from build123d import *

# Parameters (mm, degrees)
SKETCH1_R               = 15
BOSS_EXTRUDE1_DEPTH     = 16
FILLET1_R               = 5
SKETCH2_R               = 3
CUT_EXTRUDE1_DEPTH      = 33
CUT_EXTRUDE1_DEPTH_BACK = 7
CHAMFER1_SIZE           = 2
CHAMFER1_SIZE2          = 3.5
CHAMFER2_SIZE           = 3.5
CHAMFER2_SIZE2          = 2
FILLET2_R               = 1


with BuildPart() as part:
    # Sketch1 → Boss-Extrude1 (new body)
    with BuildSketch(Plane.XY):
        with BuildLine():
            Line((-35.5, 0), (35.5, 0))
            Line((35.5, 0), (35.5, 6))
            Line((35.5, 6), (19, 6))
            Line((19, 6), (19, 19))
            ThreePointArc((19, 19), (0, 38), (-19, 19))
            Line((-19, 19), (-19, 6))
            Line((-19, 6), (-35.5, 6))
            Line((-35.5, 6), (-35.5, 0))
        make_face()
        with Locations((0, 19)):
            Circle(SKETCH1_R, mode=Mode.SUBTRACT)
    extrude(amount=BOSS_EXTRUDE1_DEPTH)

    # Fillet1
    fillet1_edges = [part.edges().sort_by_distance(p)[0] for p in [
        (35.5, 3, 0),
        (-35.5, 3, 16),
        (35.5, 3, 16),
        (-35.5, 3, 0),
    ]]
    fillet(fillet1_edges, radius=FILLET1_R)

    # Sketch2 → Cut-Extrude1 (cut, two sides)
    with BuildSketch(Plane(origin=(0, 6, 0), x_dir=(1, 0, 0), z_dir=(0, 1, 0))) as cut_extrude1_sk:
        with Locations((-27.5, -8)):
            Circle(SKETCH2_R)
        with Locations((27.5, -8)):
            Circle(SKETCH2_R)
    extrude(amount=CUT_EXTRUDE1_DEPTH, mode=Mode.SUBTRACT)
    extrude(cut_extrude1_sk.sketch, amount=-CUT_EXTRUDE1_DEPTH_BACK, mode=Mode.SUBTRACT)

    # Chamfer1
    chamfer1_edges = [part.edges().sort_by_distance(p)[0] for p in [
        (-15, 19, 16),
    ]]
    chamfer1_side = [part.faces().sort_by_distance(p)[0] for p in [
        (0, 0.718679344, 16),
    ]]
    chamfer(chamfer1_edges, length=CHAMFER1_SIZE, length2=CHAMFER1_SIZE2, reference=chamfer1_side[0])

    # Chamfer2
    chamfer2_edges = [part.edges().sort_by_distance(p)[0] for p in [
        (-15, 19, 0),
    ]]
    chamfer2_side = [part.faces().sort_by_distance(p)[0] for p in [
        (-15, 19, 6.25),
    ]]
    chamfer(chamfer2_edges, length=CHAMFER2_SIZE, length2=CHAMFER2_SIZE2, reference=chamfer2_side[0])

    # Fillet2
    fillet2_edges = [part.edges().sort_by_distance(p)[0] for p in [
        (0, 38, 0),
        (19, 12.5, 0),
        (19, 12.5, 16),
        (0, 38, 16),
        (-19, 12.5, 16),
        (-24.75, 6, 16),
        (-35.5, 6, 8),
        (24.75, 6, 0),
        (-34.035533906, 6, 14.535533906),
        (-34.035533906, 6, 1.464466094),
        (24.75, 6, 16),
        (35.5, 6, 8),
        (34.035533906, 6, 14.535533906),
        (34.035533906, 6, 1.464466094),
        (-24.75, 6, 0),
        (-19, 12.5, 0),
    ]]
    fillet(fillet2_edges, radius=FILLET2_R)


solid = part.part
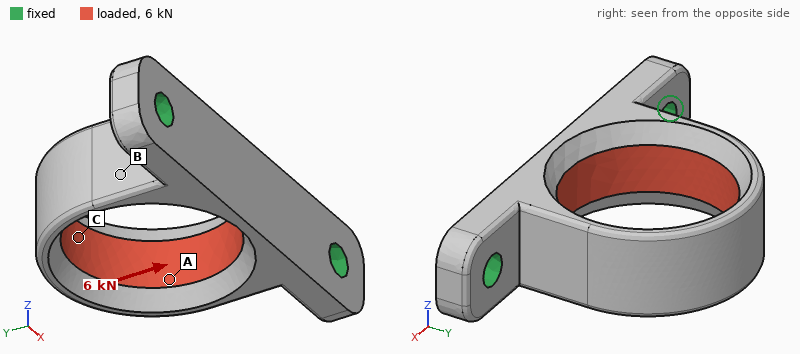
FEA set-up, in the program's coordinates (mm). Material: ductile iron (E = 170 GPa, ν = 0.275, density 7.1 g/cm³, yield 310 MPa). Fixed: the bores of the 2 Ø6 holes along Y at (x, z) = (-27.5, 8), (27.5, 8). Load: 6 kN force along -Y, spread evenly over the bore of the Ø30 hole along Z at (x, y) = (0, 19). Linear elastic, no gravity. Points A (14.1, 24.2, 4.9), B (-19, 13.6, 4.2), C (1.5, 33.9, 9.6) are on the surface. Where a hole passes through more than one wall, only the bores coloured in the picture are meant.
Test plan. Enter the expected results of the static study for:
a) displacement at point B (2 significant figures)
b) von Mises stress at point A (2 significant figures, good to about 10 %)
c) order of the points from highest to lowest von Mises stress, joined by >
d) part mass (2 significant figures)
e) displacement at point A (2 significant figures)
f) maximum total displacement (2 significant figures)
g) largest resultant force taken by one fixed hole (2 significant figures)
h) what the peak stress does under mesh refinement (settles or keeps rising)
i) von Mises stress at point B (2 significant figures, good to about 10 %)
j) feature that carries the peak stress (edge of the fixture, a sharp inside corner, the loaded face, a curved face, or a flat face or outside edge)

20 µm
57 MPa
B > A > C
80 g
18 µm
36 µm
3.0 kN
keeps rising
110 MPa
edge of the fixture
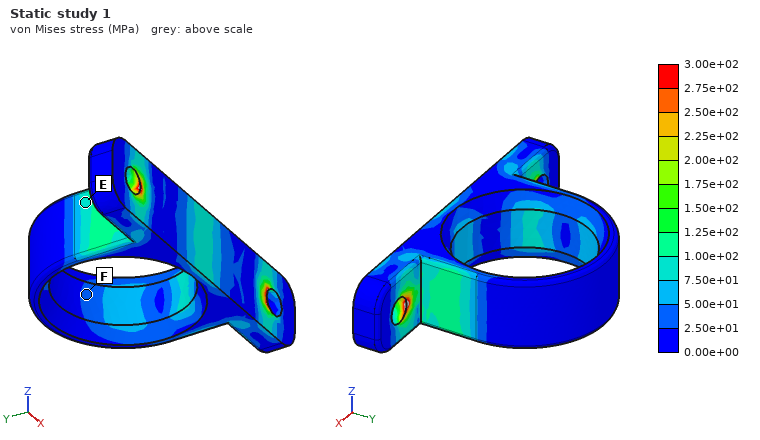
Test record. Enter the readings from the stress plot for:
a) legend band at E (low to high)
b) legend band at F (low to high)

7.50e+01 to 1.00e+02 MPa
2.50e+01 to 5.00e+01 MPa
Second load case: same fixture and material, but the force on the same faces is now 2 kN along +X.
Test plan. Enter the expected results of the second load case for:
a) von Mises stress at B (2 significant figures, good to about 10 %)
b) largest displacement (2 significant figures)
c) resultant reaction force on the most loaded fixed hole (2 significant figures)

70 MPa
43 µm
1.2 kN
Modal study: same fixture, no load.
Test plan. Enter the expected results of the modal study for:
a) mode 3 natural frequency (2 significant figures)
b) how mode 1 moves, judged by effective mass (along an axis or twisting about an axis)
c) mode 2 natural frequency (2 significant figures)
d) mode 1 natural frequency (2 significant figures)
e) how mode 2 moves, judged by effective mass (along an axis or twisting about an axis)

9000 Hz
along Z
5700 Hz
4100 Hz
along X
